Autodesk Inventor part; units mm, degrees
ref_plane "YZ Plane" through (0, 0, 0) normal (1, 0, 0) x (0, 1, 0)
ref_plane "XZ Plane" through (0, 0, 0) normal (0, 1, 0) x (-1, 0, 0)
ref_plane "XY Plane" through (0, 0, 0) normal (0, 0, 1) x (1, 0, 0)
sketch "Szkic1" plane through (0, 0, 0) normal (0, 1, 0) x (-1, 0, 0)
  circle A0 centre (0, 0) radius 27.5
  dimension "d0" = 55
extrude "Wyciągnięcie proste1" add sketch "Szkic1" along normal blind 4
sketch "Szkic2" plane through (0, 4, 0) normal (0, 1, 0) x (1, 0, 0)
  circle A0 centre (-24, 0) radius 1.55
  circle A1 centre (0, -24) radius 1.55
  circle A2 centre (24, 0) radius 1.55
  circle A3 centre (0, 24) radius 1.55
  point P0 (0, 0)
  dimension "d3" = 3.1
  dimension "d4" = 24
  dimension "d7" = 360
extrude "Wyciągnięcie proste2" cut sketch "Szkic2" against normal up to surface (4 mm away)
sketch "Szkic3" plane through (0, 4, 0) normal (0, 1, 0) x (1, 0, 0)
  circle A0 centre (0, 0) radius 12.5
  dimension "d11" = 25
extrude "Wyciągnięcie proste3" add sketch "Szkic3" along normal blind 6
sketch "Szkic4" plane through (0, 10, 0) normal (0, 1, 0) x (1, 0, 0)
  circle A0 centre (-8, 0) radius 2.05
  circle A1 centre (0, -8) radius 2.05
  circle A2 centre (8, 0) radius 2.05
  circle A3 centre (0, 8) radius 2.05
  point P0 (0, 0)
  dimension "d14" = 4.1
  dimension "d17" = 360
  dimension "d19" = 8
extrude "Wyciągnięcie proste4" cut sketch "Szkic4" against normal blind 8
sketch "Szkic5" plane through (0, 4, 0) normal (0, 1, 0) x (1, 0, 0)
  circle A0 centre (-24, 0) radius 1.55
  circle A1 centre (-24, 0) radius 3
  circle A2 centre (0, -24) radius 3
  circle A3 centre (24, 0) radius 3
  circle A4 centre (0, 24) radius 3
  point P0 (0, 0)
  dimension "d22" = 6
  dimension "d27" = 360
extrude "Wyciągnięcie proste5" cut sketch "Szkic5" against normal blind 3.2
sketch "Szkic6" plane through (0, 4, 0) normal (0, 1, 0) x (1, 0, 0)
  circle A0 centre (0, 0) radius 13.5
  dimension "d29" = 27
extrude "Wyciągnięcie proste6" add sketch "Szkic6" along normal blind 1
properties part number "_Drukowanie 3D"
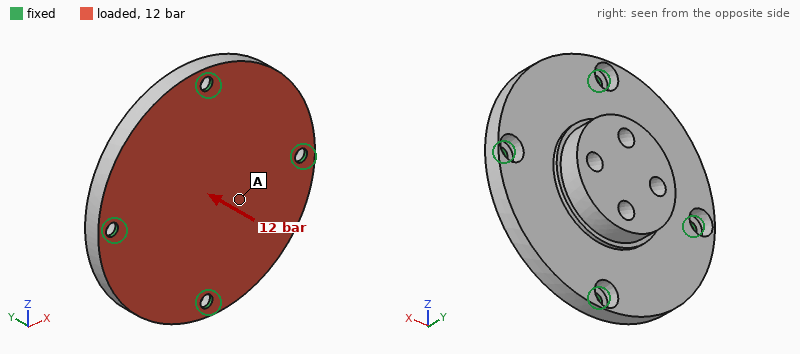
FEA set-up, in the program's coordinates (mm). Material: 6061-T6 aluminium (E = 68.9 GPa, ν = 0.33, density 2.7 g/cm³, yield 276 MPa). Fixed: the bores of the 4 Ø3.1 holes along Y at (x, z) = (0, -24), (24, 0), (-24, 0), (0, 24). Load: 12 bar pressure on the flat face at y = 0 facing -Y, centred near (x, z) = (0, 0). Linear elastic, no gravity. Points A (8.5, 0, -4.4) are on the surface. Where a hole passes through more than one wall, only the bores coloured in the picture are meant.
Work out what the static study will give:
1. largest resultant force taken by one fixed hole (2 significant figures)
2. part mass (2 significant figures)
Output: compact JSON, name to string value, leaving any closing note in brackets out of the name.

{"largest resultant force taken by one fixed hole": "880 N", "part mass": "32 g"}
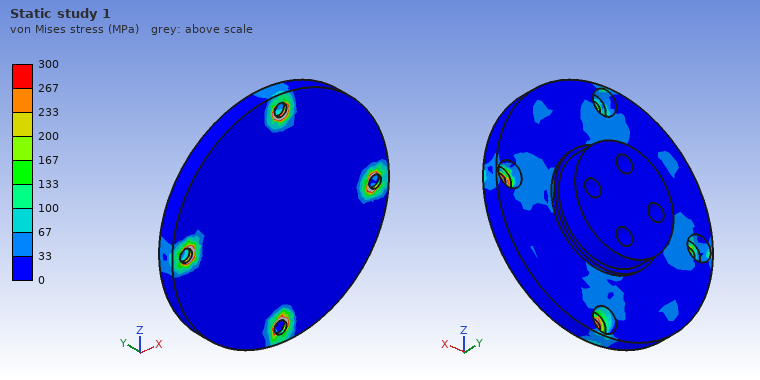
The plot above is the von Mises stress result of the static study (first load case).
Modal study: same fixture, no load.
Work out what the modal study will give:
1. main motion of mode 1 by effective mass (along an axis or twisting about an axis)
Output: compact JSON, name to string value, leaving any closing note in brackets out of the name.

{"main motion of mode 1 by effective mass": "along Y"}
